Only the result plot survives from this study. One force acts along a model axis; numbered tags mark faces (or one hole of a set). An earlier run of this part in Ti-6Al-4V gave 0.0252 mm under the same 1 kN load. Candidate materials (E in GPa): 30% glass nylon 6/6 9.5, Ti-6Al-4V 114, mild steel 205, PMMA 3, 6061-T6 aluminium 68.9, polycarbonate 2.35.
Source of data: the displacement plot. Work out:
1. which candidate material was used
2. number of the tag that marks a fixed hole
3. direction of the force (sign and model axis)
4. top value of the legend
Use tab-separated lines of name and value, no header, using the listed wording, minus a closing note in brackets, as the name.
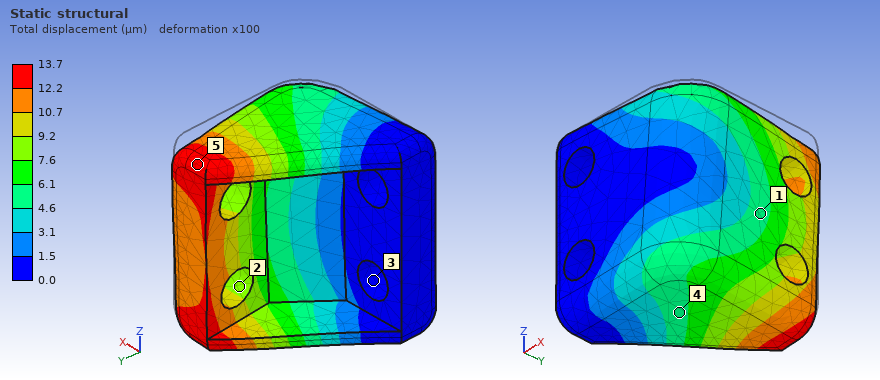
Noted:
which candidate material was used	mild steel
number of the tag that marks a fixed hole	3
direction of the force	-Z
top value of the legend	13.7 µm
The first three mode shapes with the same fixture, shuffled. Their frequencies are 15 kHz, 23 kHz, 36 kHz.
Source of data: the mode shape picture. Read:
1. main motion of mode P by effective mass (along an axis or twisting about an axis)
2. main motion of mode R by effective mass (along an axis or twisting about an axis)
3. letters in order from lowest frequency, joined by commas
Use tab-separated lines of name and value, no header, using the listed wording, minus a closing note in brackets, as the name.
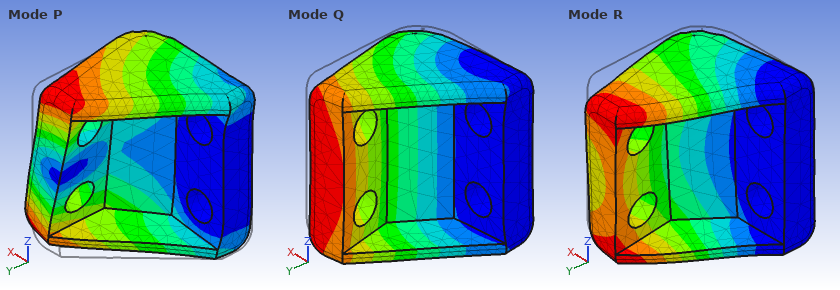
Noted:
main motion of mode P by effective mass	along Z
main motion of mode R by effective mass	along Z
letters in order from lowest frequency, joined by commas	Q, R, P
